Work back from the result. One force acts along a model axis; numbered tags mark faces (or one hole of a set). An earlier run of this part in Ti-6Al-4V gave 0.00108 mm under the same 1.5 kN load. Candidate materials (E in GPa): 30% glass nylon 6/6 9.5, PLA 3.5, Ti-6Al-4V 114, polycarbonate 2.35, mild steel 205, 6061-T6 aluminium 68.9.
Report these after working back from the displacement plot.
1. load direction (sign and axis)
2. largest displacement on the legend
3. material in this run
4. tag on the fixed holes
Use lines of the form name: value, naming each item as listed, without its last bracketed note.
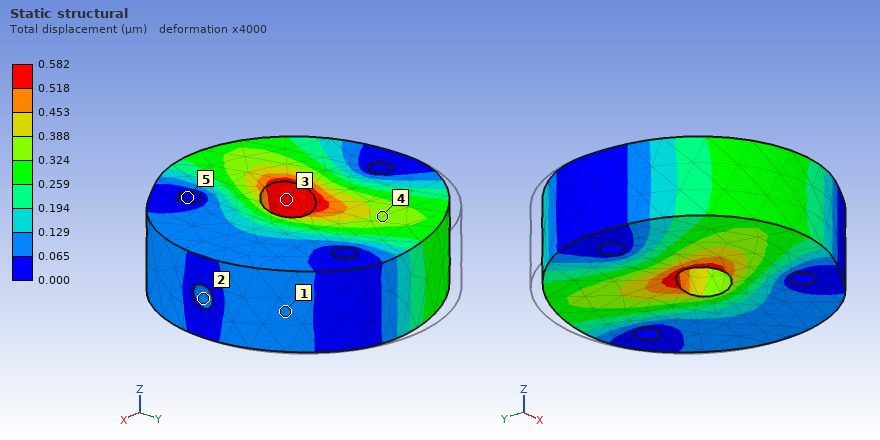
load direction: -Y
largest displacement on the legend: 0.582 µm
material in this run: mild steel
tag on the fixed holes: 5
